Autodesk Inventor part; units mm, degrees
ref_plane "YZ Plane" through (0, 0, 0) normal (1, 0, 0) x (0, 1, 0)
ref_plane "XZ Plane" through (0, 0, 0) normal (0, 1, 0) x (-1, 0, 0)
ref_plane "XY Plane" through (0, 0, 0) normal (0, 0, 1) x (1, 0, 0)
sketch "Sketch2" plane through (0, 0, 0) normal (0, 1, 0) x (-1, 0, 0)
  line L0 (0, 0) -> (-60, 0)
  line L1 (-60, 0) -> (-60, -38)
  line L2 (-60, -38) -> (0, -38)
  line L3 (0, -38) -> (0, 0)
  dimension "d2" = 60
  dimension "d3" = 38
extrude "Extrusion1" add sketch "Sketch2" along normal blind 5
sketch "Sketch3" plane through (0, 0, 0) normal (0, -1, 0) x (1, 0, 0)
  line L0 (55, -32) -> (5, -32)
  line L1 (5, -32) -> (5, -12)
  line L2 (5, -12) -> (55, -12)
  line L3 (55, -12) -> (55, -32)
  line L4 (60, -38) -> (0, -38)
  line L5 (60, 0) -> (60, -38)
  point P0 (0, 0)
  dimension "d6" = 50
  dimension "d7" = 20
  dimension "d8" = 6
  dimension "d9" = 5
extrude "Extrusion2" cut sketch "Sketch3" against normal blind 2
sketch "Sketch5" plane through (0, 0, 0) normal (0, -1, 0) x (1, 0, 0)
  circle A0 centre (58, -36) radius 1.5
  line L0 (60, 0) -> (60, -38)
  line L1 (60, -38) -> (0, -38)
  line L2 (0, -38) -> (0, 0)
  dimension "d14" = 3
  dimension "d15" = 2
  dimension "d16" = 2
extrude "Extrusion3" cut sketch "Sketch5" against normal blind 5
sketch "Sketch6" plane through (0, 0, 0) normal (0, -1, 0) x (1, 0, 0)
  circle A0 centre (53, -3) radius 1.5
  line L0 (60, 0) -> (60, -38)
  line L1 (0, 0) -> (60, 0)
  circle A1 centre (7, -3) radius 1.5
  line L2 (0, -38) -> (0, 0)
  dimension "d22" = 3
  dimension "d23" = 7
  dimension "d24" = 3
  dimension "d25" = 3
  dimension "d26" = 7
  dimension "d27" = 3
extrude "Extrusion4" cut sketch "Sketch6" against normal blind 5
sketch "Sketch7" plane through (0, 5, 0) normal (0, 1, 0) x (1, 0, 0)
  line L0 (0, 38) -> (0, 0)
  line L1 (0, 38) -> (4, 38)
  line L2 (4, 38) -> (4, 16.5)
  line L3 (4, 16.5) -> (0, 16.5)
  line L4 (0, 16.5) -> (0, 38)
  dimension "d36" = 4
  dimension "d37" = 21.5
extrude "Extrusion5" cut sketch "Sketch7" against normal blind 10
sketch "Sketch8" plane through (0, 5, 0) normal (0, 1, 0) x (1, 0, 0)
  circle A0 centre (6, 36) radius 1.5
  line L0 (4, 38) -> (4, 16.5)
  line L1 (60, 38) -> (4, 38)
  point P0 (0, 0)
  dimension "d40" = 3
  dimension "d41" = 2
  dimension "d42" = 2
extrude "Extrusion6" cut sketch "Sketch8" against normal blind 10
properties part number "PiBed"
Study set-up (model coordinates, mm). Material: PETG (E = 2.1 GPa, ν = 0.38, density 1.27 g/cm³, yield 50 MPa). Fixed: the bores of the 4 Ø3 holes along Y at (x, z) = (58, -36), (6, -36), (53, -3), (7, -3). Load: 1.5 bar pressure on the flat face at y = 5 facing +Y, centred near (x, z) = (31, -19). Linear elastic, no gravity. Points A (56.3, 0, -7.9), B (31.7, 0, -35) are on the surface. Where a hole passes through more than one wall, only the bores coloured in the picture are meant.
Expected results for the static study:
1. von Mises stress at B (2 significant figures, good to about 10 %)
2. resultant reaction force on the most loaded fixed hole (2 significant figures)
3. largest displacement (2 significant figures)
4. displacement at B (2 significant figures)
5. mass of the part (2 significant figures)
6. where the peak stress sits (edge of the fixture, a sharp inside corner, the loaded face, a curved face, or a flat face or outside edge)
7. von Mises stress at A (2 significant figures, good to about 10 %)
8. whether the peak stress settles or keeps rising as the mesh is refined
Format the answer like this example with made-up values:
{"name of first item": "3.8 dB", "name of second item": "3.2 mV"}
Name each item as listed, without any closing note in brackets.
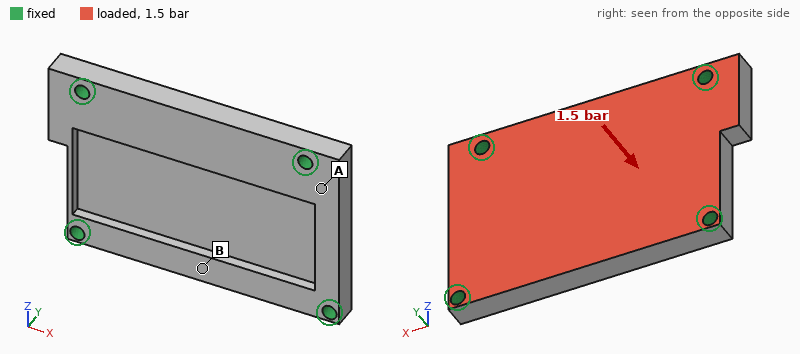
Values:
{"von Mises stress at B": "7.5 MPa", "resultant reaction force on the most loaded fixed hole": "100 N", "largest displacement": "0.29 mm", "displacement at B": "0.25 mm", "mass of the part": "11 g", "where the peak stress sits": "edge of the fixture", "von Mises stress at A": "3.5 MPa", "whether the peak stress settles or keeps rising as the mesh is refined": "keeps rising"}
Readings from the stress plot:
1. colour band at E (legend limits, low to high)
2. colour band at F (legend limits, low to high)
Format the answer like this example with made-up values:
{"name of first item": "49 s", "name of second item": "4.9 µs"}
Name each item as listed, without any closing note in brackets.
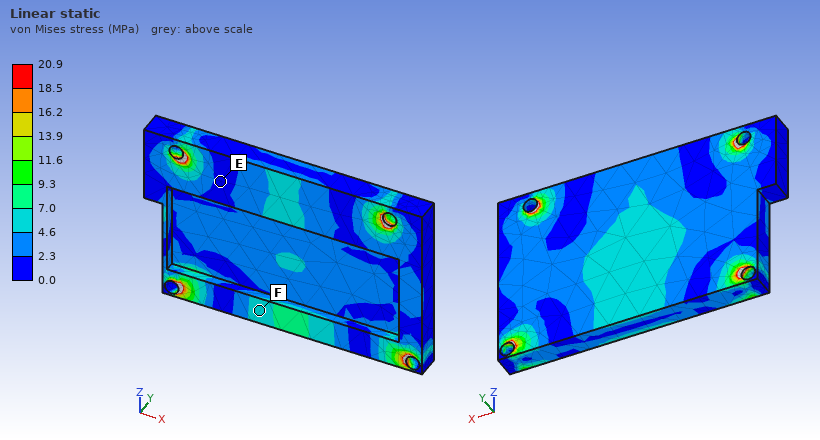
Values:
{"colour band at E": "0.0 to 2.3 MPa", "colour band at F": "4.6 to 7.0 MPa"}
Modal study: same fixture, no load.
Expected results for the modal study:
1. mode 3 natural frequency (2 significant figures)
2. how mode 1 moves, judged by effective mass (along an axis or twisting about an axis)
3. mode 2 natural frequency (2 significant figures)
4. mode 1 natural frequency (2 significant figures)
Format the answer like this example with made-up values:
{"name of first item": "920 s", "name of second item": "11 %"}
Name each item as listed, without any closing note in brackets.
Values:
{"mode 3 natural frequency": "4300 Hz", "how mode 1 moves, judged by effective mass": "along Y", "mode 2 natural frequency": "3000 Hz", "mode 1 natural frequency": "2000 Hz"}
